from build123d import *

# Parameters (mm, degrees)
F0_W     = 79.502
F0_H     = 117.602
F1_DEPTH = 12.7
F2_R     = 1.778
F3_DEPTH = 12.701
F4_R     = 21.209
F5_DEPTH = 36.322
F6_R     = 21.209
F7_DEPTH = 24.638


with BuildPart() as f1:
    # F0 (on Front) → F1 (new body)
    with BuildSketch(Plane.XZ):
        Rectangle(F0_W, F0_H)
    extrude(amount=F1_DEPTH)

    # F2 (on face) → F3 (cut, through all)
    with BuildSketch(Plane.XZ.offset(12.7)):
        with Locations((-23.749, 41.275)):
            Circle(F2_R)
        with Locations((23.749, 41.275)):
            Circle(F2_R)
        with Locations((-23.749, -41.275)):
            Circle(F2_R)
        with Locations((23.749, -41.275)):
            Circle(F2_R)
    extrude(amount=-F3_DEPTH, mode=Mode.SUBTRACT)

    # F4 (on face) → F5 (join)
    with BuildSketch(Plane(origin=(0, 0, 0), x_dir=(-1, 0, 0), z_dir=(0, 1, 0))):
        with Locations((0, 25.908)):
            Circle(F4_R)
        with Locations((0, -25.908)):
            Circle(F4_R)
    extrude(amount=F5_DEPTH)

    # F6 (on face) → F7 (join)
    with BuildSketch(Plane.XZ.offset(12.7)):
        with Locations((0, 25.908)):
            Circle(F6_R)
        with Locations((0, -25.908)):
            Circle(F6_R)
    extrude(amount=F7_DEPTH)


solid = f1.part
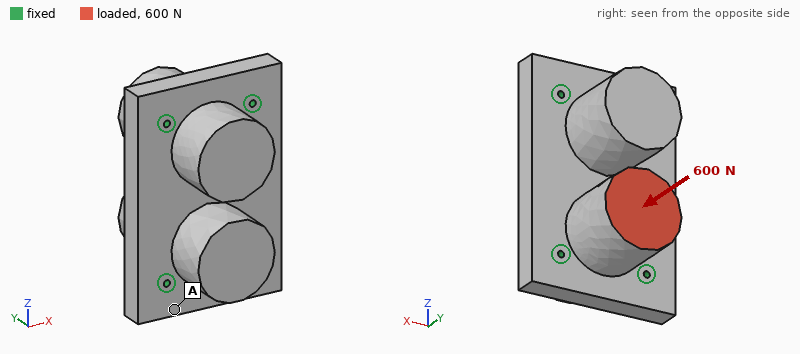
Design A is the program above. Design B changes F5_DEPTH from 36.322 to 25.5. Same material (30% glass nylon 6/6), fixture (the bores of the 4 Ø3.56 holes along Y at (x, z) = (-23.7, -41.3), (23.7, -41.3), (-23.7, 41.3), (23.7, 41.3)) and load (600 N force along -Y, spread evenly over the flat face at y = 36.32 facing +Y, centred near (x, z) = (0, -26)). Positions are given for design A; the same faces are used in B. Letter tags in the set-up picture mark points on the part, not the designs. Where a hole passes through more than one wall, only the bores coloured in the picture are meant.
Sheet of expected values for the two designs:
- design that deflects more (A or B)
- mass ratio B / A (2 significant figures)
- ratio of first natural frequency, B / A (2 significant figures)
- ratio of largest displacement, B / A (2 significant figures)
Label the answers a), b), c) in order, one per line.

a) A
b) 0.89
c) 1.2
d) 0.90
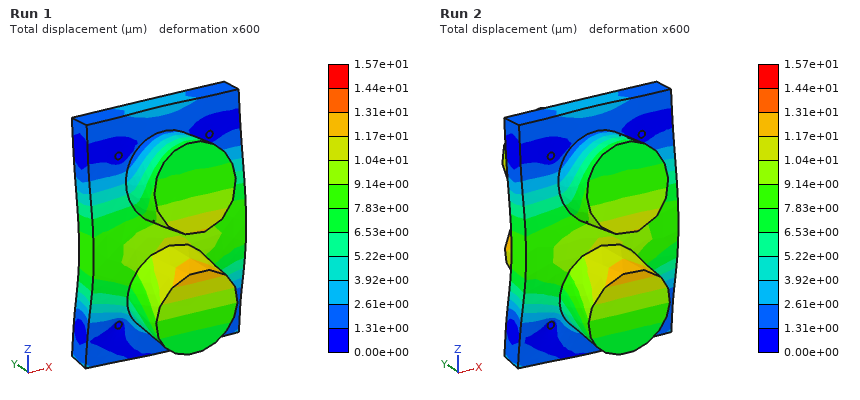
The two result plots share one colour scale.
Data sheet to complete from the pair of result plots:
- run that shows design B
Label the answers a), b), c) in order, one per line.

a) Run 1
